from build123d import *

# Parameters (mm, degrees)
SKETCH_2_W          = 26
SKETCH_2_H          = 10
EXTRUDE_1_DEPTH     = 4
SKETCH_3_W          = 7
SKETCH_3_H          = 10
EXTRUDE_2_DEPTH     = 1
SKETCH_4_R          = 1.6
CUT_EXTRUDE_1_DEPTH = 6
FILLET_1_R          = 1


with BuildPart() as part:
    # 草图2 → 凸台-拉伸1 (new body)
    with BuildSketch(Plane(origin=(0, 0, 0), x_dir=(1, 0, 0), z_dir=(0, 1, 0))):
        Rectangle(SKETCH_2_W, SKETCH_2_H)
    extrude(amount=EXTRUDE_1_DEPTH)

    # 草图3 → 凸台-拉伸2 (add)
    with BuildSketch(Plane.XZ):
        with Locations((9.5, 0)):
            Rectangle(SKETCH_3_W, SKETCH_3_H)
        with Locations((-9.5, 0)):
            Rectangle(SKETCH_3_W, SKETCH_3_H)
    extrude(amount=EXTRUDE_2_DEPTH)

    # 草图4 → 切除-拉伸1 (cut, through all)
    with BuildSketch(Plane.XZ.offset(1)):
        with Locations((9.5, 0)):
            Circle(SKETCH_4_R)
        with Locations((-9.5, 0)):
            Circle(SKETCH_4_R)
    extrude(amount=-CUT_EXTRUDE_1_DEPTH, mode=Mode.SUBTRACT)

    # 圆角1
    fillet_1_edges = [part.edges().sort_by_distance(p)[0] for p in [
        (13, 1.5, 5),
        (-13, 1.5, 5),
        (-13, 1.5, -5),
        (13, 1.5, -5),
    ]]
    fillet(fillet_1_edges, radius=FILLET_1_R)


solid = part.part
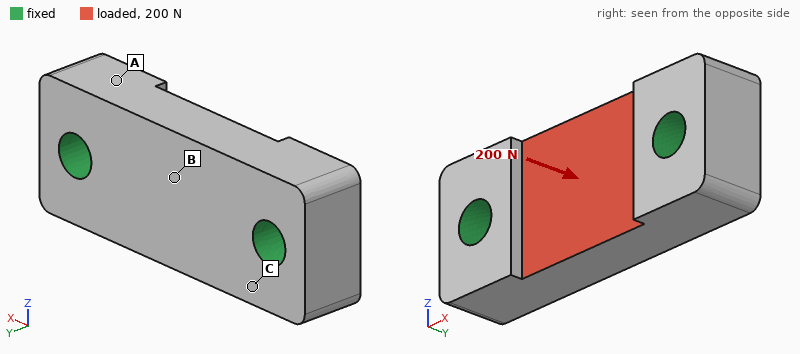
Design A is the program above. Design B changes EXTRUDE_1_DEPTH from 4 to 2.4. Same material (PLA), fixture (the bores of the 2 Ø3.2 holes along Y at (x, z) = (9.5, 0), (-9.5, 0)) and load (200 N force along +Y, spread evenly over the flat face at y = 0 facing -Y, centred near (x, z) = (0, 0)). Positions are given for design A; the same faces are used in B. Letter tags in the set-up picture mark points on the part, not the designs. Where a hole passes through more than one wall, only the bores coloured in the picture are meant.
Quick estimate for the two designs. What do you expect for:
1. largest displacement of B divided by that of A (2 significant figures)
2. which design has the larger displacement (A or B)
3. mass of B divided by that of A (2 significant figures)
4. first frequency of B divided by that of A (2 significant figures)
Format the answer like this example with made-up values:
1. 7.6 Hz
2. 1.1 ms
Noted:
1. 2.8
2. B
3. 0.64
4. 0.80
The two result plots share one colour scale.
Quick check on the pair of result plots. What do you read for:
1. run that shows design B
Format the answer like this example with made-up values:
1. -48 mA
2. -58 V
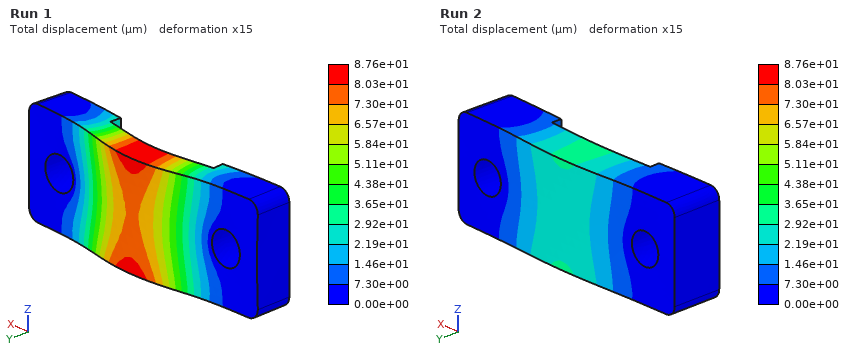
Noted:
1. Run 1
